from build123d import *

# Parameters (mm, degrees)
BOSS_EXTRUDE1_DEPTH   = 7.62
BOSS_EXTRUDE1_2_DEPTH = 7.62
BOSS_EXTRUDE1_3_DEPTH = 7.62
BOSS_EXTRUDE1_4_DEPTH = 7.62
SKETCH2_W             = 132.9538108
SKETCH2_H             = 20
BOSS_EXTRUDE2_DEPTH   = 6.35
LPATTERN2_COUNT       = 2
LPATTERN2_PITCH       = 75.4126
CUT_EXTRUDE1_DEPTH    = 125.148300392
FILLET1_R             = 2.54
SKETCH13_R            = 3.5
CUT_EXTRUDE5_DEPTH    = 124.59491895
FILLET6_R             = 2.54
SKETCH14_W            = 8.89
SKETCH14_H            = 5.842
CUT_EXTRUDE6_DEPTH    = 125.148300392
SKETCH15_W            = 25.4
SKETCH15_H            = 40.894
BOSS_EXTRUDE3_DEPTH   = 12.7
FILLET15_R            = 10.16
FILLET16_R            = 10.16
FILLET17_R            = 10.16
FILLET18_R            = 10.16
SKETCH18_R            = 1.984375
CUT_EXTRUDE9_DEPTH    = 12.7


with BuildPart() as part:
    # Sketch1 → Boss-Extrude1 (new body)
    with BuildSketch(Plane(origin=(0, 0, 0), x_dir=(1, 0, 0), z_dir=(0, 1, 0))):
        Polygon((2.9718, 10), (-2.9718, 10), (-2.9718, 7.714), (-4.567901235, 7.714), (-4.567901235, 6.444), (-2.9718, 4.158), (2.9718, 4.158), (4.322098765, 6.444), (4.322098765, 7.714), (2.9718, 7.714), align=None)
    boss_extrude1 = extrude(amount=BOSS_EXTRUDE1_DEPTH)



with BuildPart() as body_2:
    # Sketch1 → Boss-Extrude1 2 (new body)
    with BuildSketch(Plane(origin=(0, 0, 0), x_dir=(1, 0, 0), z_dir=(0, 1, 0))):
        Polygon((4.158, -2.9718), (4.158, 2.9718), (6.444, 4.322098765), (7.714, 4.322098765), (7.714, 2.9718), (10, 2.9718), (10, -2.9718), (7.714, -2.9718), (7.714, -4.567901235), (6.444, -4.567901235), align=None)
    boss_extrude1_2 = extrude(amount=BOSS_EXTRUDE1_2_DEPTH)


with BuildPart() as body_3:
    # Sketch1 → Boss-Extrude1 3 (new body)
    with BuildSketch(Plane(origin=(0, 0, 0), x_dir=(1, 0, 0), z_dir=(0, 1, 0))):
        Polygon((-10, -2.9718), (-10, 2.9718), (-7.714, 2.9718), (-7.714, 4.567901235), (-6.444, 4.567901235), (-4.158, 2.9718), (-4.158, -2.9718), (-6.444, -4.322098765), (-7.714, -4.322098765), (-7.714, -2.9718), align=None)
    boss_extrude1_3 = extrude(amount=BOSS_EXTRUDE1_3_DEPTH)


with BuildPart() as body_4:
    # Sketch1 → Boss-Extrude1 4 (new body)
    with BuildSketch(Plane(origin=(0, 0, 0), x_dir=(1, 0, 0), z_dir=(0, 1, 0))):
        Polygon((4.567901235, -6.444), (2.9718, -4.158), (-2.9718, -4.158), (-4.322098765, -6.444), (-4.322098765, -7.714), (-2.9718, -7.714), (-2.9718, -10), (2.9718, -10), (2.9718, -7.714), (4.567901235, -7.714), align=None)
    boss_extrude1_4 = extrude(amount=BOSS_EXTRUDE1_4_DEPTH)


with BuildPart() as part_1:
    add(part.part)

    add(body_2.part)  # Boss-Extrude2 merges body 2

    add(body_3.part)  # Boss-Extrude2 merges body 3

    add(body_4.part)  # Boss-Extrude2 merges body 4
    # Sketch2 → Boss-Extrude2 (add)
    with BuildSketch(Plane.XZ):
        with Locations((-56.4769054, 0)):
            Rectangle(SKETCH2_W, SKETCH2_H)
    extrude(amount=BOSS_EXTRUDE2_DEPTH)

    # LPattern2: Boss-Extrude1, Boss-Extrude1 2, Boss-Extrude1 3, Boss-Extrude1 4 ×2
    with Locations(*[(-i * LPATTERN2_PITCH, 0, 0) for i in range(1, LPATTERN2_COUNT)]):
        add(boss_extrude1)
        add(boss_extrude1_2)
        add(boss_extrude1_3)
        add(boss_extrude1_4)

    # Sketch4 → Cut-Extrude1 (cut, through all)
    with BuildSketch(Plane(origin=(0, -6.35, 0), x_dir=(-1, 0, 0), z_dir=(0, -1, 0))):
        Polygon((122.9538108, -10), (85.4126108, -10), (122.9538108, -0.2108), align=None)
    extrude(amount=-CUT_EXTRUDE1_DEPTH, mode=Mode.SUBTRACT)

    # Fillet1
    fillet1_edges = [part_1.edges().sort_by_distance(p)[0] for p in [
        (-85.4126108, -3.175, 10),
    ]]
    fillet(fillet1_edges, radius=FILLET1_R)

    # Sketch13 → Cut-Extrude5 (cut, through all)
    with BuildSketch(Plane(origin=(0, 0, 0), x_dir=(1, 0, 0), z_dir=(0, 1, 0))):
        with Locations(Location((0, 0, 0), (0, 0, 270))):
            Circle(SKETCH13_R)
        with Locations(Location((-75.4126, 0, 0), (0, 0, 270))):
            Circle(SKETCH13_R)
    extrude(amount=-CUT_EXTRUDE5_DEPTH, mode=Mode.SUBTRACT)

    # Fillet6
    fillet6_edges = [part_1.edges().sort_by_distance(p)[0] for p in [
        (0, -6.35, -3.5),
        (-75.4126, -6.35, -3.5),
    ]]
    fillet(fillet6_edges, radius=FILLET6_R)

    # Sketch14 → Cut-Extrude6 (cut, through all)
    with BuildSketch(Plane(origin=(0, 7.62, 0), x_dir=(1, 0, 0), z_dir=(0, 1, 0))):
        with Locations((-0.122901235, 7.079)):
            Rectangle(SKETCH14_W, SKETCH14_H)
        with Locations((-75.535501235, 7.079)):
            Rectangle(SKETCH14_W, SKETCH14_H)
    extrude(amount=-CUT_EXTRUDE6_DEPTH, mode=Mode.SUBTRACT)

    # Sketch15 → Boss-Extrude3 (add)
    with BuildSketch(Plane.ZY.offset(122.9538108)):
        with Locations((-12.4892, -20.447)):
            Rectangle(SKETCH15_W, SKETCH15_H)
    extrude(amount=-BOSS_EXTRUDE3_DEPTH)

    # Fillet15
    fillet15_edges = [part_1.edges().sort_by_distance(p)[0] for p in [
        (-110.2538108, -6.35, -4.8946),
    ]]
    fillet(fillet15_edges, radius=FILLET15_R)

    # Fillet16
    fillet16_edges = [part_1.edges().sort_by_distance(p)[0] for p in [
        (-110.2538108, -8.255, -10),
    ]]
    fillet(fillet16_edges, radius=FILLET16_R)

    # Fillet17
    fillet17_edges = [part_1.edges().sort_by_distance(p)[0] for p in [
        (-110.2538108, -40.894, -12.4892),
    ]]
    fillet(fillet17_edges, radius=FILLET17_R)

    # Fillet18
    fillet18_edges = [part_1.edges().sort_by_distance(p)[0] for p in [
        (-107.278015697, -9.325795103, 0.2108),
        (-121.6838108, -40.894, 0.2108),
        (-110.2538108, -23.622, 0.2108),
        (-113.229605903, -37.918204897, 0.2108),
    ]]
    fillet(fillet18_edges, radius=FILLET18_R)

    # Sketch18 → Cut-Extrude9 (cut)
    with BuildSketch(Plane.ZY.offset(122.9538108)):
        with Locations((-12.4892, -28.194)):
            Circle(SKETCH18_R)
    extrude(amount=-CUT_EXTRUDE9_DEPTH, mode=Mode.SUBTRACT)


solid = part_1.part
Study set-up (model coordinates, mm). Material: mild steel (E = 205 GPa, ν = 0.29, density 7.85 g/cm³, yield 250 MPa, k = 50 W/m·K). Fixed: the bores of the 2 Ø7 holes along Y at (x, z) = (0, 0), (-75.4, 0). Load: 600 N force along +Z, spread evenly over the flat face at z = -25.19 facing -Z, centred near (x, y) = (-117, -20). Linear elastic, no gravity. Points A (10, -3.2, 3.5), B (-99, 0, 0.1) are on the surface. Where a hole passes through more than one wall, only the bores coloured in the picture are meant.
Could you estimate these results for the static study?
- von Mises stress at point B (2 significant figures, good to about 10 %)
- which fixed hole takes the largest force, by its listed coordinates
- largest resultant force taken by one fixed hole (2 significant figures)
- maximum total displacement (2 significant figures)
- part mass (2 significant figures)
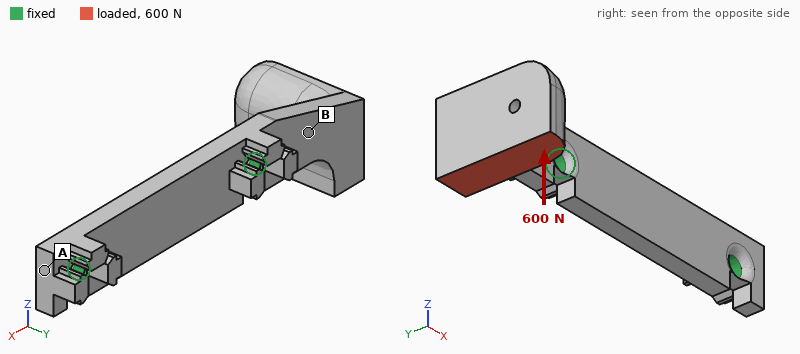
75 MPa
(-75.4, 0)
710 N
0.22 mm
220 g
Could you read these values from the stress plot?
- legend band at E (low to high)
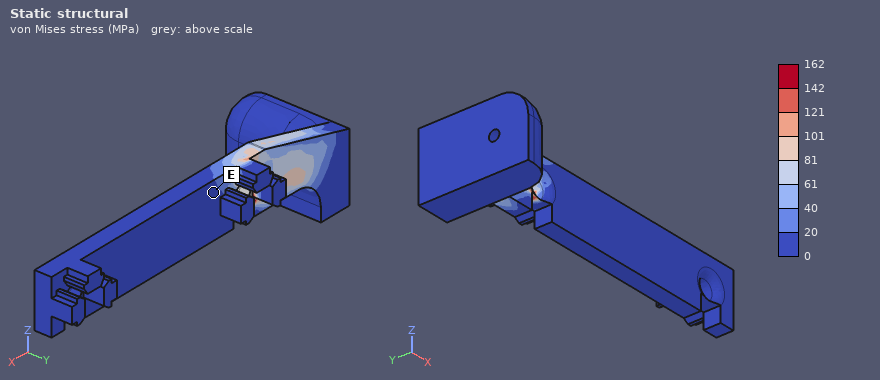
0 to 20 MPa
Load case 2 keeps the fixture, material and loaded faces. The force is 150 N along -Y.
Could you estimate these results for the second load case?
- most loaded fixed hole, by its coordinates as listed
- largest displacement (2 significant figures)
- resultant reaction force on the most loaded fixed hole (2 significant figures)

(-75.4, 0)
0.14 mm
150 N
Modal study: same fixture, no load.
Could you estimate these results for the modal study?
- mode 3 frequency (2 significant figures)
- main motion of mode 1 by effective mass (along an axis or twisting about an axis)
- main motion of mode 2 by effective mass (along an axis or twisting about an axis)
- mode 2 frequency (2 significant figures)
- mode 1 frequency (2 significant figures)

2800 Hz
along Y
along Z
1100 Hz
670 Hz
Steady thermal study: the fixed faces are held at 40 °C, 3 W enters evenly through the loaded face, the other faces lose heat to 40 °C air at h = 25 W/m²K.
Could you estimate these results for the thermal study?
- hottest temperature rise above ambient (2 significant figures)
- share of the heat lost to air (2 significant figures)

16 K
43 %
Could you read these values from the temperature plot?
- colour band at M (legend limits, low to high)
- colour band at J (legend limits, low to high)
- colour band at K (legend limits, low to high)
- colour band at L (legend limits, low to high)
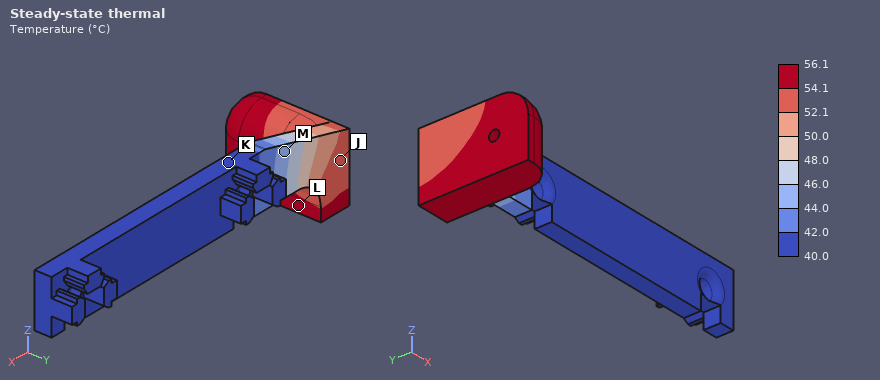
44.0 to 46.0 °C
52.1 to 54.1 °C
40.0 to 42.0 °C
54.1 to 56.1 °C
